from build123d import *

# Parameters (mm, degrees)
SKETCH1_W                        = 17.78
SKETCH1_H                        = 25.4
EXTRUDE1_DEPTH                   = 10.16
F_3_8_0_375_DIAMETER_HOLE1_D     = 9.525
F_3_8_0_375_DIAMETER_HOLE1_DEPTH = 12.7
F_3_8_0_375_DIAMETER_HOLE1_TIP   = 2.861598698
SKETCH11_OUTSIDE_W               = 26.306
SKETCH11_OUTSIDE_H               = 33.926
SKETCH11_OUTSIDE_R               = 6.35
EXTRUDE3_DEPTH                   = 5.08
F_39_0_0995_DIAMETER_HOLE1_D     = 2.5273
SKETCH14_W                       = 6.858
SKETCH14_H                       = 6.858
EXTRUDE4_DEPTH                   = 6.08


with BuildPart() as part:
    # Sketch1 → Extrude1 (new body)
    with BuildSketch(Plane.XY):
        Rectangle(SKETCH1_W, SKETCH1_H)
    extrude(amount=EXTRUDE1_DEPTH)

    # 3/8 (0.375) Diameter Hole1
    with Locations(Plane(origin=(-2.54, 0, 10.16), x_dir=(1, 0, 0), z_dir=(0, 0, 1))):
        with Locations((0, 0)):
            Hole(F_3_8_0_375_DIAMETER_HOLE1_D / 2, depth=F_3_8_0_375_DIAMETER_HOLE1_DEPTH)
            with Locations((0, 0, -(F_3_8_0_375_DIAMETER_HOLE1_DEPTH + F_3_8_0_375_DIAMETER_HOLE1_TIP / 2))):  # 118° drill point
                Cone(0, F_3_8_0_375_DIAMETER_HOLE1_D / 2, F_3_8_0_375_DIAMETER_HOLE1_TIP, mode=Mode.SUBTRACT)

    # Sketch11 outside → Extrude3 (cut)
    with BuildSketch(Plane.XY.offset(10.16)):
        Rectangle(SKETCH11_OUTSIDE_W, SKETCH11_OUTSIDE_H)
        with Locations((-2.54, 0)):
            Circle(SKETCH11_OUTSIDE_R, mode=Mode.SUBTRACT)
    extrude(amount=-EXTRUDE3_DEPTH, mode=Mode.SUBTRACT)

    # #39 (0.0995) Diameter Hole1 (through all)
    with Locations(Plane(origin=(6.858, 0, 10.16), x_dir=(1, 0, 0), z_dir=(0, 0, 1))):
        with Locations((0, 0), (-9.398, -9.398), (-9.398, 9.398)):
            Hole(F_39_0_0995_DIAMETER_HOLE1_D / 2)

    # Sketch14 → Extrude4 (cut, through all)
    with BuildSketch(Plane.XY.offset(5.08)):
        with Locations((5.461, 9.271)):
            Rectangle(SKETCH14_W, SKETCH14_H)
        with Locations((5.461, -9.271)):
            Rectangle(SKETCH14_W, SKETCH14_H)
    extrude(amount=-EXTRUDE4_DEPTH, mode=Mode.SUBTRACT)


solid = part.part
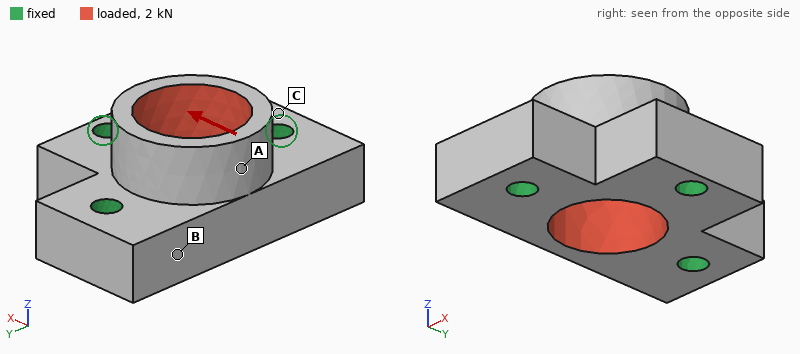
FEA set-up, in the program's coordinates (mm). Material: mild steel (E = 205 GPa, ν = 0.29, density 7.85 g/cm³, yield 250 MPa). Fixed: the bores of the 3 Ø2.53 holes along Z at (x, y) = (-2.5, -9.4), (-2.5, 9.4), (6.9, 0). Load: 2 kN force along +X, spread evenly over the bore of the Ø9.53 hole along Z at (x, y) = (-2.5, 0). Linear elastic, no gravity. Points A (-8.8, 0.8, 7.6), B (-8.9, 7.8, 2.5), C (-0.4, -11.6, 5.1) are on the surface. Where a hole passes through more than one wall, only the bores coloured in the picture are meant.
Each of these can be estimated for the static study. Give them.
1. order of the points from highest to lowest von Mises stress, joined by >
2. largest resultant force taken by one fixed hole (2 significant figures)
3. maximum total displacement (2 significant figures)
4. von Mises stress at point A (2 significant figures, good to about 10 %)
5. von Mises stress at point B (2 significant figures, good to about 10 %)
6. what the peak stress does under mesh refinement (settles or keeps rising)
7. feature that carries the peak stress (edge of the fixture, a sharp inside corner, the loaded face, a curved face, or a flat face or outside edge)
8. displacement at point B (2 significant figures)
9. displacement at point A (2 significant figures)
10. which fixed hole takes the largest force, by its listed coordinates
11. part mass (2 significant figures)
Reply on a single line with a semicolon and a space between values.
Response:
A > B > C; 840 N; 7.0 µm; 36 MPa; 19 MPa; keeps rising; edge of the fixture; 1.4 µm; 5.6 µm; (6.9, 0); 13 g
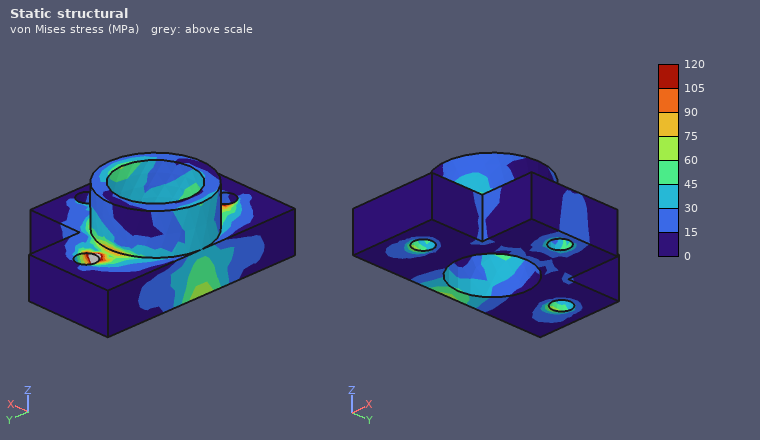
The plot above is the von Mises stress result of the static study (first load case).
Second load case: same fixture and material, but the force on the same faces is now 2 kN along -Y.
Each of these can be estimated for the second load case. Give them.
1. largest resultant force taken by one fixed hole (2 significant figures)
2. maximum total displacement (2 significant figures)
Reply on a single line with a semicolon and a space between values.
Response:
870 N; 3.1 µm
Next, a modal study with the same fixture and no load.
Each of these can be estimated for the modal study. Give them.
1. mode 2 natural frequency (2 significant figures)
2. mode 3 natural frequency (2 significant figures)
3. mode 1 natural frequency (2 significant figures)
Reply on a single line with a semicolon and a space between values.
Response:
54 kHz; 70 kHz; 40 kHz
